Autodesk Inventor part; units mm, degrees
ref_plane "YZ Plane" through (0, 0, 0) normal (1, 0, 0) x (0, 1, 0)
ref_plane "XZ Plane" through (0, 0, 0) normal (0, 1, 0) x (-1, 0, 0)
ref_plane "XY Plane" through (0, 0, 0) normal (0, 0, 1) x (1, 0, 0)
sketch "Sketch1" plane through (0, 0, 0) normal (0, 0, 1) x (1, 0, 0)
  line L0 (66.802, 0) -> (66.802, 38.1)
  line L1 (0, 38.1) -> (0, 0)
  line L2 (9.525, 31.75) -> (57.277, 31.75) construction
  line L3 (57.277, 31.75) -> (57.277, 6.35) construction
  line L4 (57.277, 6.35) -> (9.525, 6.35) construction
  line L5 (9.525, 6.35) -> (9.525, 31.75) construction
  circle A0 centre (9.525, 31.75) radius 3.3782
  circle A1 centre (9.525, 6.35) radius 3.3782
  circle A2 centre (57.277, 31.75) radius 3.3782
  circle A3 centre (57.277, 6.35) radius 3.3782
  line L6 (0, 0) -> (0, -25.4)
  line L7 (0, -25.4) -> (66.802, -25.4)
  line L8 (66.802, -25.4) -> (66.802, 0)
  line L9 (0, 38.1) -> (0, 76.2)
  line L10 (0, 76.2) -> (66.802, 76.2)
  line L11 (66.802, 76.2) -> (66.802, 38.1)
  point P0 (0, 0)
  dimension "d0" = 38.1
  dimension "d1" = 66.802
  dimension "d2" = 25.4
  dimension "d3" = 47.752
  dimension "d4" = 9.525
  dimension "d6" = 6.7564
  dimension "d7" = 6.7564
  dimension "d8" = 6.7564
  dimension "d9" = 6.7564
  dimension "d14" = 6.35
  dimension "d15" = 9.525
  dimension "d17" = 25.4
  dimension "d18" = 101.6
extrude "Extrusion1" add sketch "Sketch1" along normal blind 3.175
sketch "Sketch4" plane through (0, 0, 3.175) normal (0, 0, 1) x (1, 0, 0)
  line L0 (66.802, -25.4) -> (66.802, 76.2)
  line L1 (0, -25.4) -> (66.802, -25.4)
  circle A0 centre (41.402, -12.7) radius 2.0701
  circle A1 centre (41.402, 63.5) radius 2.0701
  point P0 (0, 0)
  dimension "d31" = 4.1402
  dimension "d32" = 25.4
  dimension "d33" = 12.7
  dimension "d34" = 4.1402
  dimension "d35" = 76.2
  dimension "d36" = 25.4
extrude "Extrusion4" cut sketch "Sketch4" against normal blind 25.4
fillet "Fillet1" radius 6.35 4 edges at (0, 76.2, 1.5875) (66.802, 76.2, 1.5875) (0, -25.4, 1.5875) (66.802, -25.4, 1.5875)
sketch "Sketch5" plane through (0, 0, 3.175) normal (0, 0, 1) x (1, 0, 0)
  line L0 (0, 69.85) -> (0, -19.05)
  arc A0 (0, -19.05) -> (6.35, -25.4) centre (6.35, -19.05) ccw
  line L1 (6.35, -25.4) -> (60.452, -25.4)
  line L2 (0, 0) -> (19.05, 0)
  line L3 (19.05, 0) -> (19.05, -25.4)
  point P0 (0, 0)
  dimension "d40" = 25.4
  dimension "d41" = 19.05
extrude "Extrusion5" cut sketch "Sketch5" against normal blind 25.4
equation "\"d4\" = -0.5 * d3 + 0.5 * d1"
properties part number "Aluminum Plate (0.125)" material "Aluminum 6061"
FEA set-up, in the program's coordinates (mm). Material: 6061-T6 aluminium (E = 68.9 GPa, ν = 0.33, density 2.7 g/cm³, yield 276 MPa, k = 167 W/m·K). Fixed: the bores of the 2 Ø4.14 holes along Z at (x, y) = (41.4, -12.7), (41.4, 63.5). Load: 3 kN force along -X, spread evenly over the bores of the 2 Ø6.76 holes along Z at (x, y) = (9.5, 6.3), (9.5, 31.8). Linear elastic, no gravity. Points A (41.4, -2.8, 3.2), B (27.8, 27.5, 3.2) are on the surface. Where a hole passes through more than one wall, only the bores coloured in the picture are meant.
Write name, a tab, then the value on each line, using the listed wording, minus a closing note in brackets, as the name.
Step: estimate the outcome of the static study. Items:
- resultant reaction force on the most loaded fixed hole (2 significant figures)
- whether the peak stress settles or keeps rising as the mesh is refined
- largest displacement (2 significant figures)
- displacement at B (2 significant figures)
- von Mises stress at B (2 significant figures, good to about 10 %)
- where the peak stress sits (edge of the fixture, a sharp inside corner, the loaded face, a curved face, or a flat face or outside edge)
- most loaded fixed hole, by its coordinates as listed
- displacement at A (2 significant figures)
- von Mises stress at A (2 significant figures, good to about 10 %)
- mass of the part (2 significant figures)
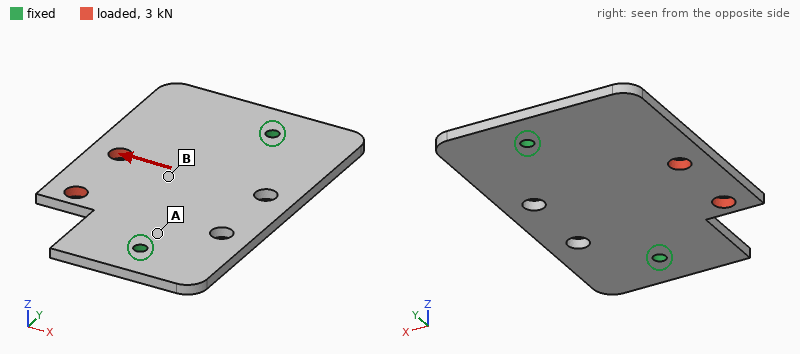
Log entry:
resultant reaction force on the most loaded fixed hole	1.8 kN
whether the peak stress settles or keeps rising as the mesh is refined	keeps rising
largest displacement	28 µm
displacement at B	17 µm
von Mises stress at B	9.8 MPa
where the peak stress sits	edge of the fixture
most loaded fixed hole, by its coordinates as listed	(41.4, -12.7)
displacement at A	8.9 µm
von Mises stress at A	23 MPa
mass of the part	52 g
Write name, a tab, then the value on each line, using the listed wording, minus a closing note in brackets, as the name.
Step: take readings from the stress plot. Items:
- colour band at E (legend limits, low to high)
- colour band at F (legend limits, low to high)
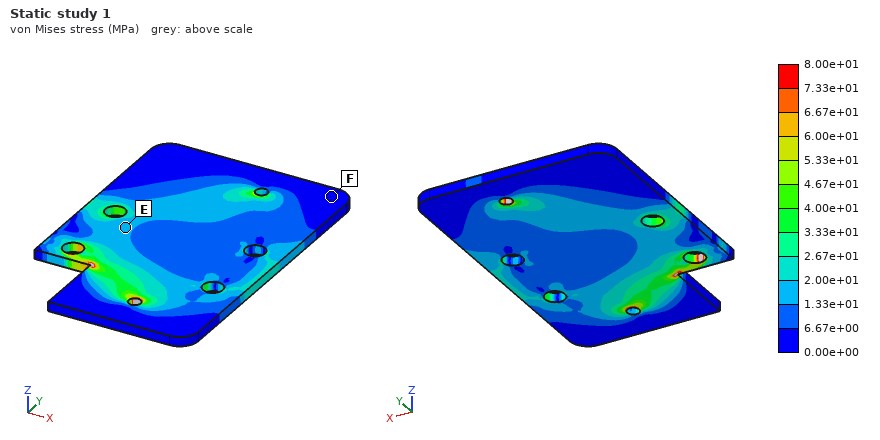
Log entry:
colour band at E	1.33e+01 to 2.00e+01 MPa
colour band at F	0.00e+00 to 6.67e+00 MPa
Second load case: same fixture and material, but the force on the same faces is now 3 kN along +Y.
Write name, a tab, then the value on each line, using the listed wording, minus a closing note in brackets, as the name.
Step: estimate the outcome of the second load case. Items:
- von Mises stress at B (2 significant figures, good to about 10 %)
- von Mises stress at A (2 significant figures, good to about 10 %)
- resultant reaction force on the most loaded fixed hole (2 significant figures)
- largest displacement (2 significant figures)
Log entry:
von Mises stress at B	18 MPa
von Mises stress at A	21 MPa
resultant reaction force on the most loaded fixed hole	1.9 kN
largest displacement	34 µm
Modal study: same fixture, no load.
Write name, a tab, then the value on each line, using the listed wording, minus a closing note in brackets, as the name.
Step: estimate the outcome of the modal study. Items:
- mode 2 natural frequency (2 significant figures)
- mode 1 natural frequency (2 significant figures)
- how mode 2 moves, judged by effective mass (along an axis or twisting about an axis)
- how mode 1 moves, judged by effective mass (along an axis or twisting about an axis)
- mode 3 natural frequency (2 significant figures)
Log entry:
mode 2 natural frequency	2200 Hz
mode 1 natural frequency	1200 Hz
how mode 2 moves, judged by effective mass	along Z
how mode 1 moves, judged by effective mass	along Z
mode 3 natural frequency	2500 Hz
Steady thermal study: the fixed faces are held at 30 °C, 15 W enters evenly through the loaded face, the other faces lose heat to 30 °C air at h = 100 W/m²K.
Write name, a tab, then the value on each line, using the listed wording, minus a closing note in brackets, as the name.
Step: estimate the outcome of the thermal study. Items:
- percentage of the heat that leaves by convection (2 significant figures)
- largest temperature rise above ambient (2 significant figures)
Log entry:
percentage of the heat that leaves by convection	45 %
largest temperature rise above ambient	19 K
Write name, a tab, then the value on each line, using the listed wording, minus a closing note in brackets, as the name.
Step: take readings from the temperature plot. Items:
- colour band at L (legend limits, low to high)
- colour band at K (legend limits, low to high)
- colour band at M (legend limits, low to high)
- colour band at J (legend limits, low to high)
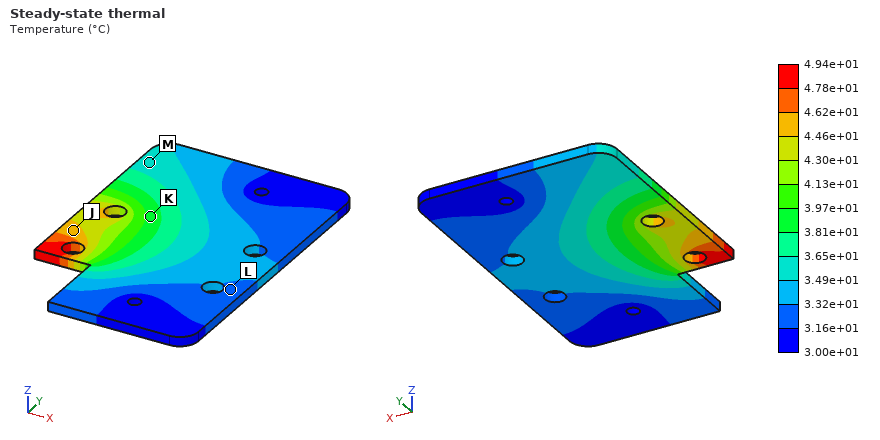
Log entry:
colour band at L	3.16e+01 to 3.32e+01 °C
colour band at K	3.81e+01 to 3.97e+01 °C
colour band at M	3.49e+01 to 3.65e+01 °C
colour band at J	4.46e+01 to 4.62e+01 °C
